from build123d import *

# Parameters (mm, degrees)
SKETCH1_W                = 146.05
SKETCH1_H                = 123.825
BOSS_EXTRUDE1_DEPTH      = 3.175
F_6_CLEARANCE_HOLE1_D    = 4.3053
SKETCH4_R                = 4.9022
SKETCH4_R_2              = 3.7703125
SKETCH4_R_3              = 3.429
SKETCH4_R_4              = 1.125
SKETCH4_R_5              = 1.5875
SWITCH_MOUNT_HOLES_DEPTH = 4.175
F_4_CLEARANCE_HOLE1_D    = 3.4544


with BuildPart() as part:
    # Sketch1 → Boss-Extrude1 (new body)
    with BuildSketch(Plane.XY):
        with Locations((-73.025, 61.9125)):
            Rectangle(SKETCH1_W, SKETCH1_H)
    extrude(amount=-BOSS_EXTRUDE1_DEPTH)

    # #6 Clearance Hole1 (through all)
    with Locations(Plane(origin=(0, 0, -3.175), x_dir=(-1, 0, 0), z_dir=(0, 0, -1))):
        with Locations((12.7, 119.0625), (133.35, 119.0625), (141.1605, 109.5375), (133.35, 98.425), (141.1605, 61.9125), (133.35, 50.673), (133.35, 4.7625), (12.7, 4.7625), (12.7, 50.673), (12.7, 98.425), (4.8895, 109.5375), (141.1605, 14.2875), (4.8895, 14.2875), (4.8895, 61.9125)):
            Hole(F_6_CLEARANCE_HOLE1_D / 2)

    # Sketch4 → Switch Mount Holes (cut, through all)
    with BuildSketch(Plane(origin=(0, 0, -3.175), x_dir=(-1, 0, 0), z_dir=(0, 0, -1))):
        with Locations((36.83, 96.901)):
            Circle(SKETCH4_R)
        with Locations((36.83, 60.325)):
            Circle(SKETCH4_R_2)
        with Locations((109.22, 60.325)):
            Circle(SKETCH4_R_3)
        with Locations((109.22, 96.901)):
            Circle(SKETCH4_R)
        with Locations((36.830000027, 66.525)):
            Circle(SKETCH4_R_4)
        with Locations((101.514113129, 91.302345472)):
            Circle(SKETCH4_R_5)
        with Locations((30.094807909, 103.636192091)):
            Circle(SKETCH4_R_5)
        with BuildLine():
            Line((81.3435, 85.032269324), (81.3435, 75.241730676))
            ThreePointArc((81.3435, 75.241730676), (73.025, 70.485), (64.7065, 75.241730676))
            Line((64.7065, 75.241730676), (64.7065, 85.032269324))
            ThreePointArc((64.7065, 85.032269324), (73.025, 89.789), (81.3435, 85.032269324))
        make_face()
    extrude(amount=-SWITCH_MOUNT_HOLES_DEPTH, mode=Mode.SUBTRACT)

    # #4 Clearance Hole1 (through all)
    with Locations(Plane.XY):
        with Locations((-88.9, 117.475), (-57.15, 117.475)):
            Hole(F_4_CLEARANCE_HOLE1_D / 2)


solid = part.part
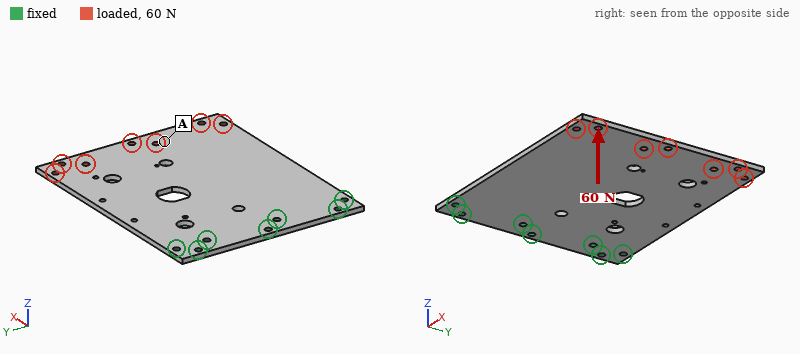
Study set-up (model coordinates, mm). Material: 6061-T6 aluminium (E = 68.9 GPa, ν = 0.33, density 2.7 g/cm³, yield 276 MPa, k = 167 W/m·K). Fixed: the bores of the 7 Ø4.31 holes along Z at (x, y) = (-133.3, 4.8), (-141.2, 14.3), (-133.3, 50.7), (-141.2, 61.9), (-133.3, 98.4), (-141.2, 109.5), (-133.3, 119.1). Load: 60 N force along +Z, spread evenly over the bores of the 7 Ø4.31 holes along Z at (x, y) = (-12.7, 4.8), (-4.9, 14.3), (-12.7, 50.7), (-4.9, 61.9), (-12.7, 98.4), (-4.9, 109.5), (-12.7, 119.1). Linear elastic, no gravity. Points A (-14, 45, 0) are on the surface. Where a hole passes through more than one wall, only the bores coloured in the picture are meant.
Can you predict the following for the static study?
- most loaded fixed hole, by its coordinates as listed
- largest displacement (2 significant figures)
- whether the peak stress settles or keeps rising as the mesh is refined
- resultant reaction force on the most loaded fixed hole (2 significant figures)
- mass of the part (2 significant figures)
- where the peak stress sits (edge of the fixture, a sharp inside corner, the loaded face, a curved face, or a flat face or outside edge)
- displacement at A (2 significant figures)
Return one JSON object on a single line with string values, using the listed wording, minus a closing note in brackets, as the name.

{"most loaded fixed hole, by its coordinates as listed": "(-133.3, 50.7)", "largest displacement": "2.0 mm", "whether the peak stress settles or keeps rising as the mesh is refined": "keeps rising", "resultant reaction force on the most loaded fixed hole": "120 N", "mass of the part": "150 g", "where the peak stress sits": "edge of the fixture", "displacement at A": "1.7 mm"}
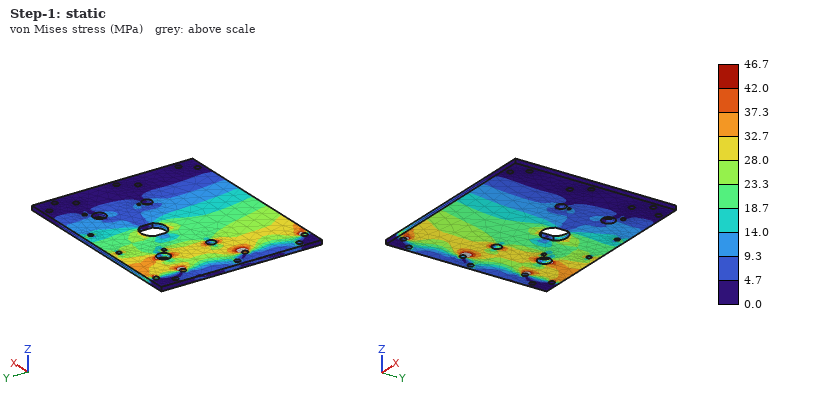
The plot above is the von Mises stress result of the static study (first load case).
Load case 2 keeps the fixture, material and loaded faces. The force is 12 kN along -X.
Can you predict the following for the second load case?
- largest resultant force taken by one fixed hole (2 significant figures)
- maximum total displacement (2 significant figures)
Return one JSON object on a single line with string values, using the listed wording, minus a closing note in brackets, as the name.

{"largest resultant force taken by one fixed hole": "2.5 kN", "maximum total displacement": "95 µm"}
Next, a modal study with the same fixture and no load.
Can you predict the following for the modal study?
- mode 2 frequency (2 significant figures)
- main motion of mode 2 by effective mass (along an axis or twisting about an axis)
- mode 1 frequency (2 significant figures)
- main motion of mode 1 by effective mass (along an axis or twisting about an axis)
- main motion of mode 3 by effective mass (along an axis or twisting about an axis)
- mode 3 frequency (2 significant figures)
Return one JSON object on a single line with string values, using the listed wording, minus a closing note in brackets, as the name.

{"mode 2 frequency": "380 Hz", "main motion of mode 2 by effective mass": "twisting about X", "mode 1 frequency": "150 Hz", "main motion of mode 1 by effective mass": "along Z", "main motion of mode 3 by effective mass": "along Z", "mode 3 frequency": "890 Hz"}
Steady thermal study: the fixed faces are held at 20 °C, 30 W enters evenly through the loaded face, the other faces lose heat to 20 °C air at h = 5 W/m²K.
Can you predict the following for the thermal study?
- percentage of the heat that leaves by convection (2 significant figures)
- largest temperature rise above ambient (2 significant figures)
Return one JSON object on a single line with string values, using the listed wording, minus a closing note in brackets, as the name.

{"percentage of the heat that leaves by convection": "17 %", "largest temperature rise above ambient": "63 K"}
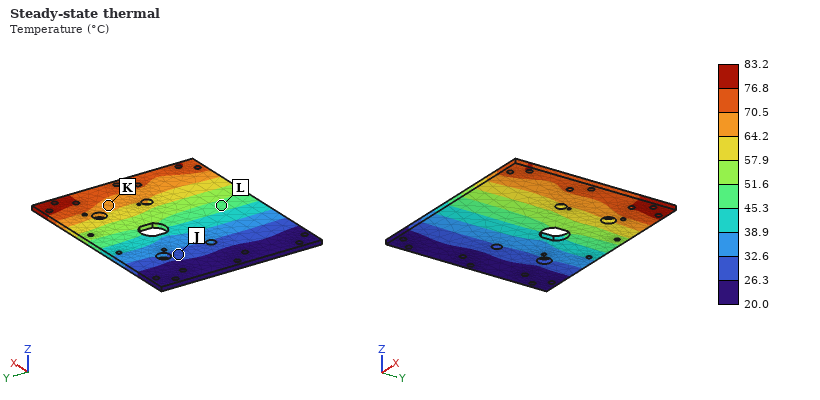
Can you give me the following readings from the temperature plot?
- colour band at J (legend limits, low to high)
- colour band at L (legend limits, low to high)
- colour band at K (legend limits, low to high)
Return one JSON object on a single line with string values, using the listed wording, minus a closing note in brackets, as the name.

{"colour band at J": "26.3 to 32.6 °C", "colour band at L": "45.3 to 51.6 °C", "colour band at K": "64.2 to 70.5 °C"}
